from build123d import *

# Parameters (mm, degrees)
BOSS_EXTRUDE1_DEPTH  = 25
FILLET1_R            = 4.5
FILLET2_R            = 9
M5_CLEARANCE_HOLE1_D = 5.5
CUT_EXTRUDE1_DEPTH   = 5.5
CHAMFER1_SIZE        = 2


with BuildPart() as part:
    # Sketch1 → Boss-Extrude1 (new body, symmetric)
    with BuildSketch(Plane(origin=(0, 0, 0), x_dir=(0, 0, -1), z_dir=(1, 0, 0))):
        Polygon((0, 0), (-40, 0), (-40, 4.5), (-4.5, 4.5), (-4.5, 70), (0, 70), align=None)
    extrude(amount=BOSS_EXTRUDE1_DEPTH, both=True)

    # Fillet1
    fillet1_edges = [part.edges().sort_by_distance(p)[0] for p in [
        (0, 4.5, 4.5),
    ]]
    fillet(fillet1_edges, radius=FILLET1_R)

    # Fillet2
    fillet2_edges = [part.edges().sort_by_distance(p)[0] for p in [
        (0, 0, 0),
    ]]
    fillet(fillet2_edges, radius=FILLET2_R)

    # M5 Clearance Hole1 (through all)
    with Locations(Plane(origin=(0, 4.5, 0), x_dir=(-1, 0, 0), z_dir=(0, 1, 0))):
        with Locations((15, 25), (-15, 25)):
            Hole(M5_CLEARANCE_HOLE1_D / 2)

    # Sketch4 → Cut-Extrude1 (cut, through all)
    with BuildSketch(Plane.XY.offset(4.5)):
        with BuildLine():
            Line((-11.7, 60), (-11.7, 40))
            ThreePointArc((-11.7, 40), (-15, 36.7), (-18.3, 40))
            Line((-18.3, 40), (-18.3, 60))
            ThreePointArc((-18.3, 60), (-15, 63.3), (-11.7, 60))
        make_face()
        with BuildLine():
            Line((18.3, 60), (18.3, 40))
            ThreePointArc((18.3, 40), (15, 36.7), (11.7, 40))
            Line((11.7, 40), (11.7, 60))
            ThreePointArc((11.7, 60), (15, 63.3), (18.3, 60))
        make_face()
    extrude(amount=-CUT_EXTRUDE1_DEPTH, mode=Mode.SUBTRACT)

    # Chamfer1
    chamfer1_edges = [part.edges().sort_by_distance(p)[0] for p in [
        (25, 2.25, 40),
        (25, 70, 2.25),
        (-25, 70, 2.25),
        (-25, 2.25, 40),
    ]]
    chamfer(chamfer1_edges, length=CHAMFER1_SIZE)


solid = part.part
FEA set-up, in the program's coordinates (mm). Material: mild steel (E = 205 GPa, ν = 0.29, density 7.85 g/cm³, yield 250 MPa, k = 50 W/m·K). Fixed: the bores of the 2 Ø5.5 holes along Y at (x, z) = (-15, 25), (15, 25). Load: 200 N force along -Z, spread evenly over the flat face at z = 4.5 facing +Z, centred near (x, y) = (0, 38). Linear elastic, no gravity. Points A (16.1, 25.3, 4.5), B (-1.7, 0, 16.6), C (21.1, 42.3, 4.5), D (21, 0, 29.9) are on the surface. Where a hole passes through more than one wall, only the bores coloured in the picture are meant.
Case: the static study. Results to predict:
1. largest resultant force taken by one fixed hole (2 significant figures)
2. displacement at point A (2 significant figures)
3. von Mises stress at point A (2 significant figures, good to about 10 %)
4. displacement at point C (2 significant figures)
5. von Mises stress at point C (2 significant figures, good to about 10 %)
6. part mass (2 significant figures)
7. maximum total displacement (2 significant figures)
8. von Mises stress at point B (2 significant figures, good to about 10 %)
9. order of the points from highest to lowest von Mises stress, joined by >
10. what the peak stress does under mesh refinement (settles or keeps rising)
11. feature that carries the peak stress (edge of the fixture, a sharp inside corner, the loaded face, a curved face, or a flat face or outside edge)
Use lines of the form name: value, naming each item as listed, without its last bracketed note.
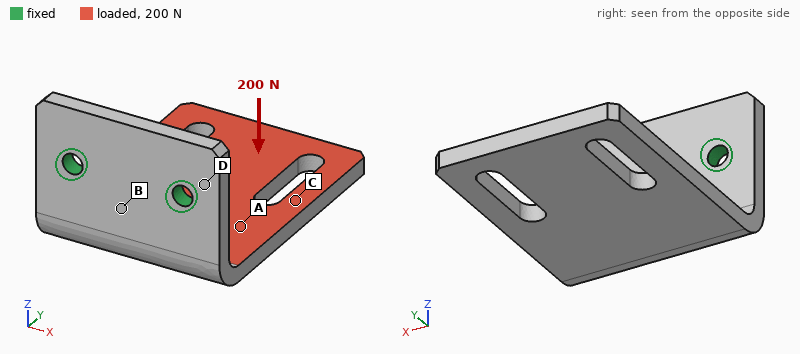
largest resultant force taken by one fixed hole: 110 N
displacement at point A: 0.060 mm
von Mises stress at point A: 17 MPa
displacement at point C: 0.12 mm
von Mises stress at point C: 11 MPa
part mass: 170 g
maximum total displacement: 0.22 mm
von Mises stress at point B: 33 MPa
order of the points from highest to lowest von Mises stress, joined by >: B > A > C > D
what the peak stress does under mesh refinement: keeps rising
feature that carries the peak stress: edge of the fixture
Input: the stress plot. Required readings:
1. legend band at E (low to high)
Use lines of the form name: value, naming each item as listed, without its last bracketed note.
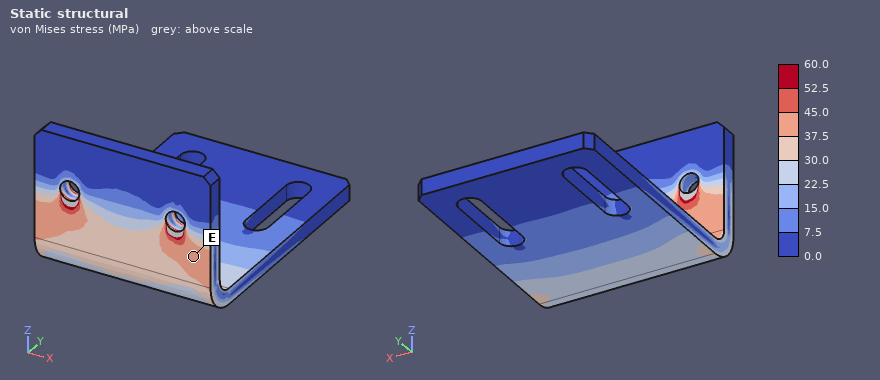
legend band at E: 37.5 to 45.0 MPa
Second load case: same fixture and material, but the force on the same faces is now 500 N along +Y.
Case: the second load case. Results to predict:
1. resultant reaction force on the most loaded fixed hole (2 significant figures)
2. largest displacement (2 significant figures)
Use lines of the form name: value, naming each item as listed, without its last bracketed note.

resultant reaction force on the most loaded fixed hole: 250 N
largest displacement: 69 µm
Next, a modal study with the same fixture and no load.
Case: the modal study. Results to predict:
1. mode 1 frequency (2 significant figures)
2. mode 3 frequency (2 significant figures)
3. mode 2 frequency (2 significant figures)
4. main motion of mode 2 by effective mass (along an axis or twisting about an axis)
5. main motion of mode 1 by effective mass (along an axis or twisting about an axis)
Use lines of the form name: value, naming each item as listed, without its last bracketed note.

mode 1 frequency: 600 Hz
mode 3 frequency: 2500 Hz
mode 2 frequency: 1400 Hz
main motion of mode 2 by effective mass: along X
main motion of mode 1 by effective mass: along Z
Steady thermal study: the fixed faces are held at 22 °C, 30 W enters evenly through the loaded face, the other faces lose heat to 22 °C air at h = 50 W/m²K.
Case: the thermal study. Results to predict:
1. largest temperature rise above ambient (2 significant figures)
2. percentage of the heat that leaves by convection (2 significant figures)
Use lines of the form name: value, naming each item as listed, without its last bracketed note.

largest temperature rise above ambient: 78 K
percentage of the heat that leaves by convection: 53 %
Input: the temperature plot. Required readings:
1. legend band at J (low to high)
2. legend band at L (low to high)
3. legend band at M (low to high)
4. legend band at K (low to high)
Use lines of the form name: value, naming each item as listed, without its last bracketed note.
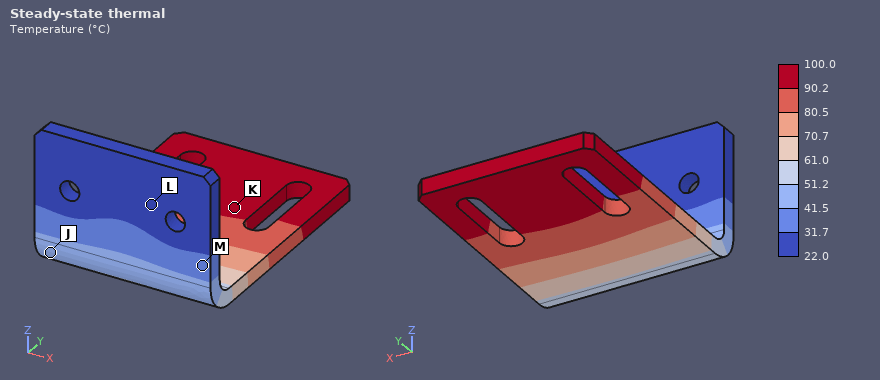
legend band at J: 41.5 to 51.2 °C
legend band at L: 22.0 to 31.7 °C
legend band at M: 31.7 to 41.5 °C
legend band at K: 90.2 to 100.0 °C
